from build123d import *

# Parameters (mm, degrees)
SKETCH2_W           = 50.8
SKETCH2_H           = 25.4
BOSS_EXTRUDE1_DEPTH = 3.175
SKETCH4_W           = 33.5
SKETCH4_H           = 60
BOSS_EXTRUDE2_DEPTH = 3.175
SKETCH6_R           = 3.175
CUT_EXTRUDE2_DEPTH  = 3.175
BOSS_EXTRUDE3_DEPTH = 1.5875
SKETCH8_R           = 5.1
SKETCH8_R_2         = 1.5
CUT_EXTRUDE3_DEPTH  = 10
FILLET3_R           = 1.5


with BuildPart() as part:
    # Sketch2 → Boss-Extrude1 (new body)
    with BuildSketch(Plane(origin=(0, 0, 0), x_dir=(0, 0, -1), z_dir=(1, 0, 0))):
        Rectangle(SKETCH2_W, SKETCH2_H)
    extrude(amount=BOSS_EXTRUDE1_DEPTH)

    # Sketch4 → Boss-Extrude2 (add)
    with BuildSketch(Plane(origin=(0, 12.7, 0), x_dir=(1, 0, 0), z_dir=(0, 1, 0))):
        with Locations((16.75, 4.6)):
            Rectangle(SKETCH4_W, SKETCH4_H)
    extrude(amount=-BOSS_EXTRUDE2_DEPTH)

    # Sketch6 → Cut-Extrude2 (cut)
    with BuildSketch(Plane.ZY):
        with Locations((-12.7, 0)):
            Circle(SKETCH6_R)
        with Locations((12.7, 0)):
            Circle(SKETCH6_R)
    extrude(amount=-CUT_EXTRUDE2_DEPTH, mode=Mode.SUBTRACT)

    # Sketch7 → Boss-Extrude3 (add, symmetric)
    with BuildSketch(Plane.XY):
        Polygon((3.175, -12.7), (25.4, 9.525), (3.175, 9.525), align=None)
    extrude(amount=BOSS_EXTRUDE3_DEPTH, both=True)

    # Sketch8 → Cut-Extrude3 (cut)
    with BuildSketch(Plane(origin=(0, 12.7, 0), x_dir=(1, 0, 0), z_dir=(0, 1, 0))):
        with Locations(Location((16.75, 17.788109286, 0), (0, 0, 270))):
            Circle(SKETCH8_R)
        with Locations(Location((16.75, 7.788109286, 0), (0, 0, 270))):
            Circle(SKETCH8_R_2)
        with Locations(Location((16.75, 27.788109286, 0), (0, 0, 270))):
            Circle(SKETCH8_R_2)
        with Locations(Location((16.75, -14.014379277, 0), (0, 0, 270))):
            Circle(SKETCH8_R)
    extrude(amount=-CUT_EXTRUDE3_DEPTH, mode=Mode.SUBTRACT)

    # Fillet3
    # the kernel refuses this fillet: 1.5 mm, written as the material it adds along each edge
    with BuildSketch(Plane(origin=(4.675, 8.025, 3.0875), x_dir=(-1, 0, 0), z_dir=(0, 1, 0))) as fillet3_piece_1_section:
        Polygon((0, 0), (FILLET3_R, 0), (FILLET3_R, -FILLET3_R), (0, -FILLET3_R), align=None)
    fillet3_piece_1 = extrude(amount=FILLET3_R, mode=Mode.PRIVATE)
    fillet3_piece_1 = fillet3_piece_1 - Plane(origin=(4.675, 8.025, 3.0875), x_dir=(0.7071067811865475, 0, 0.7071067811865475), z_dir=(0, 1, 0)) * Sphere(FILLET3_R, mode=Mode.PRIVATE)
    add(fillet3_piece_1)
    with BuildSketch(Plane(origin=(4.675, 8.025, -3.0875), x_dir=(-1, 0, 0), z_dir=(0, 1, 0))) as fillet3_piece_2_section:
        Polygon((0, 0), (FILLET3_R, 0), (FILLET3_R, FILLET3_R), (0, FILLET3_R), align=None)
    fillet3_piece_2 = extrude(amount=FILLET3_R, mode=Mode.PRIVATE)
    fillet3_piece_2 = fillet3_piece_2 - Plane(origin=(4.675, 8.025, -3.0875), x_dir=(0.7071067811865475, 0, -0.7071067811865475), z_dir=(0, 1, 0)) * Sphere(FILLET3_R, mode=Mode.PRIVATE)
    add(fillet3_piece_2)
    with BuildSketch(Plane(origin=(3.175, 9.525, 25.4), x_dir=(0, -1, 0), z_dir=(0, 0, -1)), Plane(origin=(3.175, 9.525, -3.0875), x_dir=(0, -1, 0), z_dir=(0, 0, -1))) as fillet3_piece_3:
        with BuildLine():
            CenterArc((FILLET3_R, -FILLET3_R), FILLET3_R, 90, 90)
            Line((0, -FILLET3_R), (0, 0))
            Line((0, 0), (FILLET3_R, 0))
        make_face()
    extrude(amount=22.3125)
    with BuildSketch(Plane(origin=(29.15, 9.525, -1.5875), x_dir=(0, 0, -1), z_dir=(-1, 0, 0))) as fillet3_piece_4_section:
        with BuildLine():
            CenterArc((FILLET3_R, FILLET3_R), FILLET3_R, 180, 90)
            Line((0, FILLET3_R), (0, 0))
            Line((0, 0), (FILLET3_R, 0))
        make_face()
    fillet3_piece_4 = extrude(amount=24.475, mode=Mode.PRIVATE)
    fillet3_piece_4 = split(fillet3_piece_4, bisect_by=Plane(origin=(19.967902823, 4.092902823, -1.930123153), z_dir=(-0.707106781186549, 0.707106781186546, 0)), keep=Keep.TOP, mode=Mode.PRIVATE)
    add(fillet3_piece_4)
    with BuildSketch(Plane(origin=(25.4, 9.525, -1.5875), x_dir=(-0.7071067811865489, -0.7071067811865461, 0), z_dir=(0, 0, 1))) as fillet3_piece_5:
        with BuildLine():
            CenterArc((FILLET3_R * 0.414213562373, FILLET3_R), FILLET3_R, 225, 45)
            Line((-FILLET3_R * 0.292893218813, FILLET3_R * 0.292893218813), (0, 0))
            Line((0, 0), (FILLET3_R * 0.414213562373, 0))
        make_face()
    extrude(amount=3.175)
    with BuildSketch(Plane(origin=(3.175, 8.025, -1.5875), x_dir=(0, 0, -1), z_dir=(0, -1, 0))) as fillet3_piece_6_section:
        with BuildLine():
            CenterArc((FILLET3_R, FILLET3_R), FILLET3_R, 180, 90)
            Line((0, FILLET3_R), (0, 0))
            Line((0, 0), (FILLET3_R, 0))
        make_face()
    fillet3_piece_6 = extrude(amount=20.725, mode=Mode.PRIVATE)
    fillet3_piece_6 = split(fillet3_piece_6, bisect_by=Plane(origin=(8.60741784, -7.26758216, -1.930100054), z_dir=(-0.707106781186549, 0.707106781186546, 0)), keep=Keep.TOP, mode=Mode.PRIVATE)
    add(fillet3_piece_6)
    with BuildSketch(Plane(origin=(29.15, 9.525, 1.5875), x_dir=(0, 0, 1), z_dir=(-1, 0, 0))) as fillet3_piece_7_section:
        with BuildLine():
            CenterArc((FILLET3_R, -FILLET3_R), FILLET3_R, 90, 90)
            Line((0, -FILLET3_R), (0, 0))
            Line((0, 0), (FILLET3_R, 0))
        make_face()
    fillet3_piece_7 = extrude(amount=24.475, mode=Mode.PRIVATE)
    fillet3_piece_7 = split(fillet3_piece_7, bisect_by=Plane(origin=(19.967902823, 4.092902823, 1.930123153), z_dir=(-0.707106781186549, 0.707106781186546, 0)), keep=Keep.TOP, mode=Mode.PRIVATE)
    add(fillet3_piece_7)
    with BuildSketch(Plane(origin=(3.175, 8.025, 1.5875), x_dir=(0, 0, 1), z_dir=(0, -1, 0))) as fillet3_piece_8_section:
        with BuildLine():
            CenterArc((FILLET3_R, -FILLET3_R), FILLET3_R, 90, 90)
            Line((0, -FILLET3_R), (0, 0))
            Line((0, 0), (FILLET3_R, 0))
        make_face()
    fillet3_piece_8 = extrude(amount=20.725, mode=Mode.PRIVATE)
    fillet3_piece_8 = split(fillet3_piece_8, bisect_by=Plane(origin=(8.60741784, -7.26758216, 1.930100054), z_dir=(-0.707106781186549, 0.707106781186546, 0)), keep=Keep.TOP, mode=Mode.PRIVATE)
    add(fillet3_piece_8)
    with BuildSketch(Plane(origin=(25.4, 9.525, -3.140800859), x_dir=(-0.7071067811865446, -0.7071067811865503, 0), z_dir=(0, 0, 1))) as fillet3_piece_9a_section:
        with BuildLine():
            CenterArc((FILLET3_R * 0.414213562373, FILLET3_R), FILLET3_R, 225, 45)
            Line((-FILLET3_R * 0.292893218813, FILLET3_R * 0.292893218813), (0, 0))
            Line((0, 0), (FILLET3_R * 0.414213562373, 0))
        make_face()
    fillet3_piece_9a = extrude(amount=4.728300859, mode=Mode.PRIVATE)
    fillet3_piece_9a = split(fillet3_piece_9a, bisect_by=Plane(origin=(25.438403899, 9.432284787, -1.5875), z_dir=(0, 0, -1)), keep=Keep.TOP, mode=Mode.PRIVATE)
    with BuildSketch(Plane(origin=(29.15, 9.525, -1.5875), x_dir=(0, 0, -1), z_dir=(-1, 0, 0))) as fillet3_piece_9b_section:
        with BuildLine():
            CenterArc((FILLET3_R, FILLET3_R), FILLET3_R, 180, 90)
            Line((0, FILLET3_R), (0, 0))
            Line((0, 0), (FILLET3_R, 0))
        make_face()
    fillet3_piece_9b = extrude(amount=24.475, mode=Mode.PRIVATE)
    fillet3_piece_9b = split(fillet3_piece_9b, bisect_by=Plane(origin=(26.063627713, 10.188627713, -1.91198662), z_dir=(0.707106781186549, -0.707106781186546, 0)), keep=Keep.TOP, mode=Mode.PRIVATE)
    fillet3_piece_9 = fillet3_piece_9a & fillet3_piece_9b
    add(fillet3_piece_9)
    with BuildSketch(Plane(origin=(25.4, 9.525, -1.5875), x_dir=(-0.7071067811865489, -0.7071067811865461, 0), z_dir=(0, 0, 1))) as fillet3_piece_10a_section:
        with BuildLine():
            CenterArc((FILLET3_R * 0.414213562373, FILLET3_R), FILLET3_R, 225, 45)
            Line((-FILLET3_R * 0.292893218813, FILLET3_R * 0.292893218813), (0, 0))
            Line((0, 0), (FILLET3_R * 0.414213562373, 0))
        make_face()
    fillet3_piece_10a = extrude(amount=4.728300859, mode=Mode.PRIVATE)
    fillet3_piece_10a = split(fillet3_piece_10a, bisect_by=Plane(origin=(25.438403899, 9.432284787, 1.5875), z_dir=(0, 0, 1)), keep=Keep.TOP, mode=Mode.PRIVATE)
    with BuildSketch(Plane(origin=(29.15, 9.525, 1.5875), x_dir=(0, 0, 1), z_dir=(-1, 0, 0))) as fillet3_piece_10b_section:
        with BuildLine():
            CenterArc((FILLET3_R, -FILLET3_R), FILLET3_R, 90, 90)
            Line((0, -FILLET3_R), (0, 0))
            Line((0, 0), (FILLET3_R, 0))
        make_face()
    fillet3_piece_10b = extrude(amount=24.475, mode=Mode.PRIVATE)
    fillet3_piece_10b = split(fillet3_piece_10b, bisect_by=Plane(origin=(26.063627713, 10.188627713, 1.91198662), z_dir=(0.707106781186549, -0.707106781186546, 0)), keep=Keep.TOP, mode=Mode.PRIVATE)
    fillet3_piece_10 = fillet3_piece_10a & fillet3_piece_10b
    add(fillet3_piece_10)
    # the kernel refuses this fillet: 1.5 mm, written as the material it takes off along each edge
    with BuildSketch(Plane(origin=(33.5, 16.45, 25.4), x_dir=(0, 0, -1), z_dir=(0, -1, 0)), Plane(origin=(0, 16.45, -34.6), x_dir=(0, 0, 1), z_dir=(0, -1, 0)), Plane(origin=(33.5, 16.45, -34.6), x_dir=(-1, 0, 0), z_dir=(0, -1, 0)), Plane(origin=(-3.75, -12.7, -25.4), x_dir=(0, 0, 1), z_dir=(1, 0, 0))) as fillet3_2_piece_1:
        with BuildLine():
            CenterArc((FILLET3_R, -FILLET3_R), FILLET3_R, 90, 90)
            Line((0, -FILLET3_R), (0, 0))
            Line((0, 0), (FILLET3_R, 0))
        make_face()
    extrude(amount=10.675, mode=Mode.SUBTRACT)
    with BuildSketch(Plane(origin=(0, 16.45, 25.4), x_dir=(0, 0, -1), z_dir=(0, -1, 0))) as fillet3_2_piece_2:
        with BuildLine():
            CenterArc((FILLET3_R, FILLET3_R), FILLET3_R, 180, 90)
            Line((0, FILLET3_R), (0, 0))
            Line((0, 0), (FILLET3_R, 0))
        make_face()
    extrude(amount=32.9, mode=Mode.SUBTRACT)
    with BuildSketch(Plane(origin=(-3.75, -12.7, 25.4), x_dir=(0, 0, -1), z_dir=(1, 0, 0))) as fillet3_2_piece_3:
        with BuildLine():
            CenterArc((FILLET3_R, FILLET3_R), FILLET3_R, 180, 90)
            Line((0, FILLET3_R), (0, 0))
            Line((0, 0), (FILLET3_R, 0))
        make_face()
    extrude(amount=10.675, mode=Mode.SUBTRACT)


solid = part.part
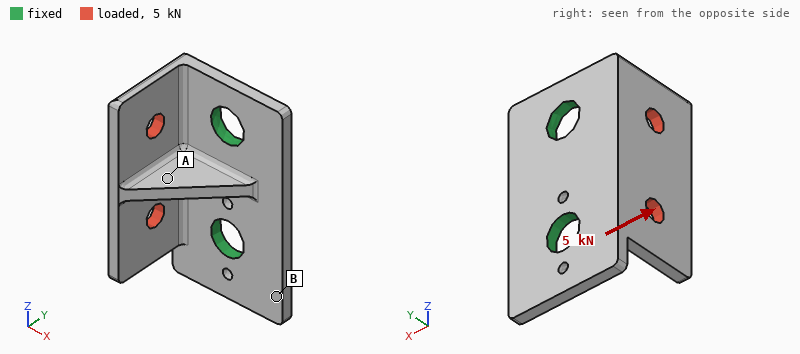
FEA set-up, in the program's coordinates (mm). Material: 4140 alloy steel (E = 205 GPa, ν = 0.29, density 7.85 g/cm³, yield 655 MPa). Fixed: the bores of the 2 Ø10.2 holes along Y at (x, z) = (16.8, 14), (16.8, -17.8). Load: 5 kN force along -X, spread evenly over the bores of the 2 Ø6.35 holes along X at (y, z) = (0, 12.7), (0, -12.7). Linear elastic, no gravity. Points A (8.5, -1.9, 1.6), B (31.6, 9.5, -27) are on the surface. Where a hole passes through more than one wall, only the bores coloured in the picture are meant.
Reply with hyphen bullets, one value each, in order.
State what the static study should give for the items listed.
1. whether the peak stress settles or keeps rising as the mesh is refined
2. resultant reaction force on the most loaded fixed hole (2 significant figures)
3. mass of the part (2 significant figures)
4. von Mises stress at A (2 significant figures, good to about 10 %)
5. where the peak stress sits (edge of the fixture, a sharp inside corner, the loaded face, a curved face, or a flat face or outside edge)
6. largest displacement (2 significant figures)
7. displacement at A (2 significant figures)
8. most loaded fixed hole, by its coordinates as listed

- keeps rising
- 2.8 kN
- 79 g
- 110 MPa
- edge of the fixture
- 0.23 mm
- 0.076 mm
- (16.8, 14)
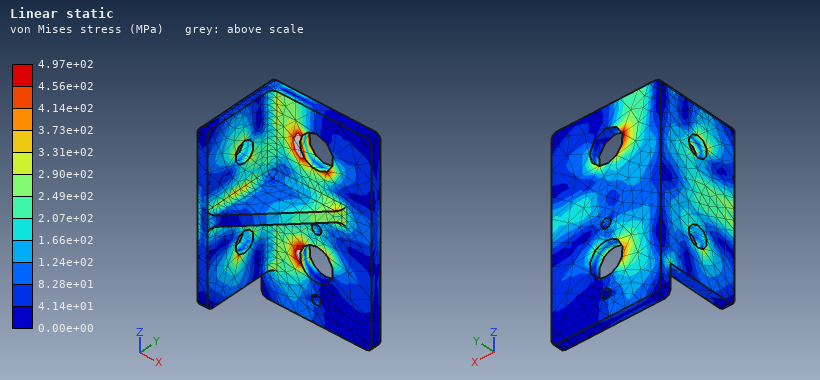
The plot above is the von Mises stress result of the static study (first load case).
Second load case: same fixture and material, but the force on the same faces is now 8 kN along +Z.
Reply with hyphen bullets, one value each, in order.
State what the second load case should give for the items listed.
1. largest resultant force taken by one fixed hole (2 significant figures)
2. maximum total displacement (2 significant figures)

- 5.5 kN
- 0.14 mm
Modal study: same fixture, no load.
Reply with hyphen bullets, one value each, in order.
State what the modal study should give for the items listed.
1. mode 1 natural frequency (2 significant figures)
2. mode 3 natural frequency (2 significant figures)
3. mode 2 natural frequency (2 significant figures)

- 4600 Hz
- 8400 Hz
- 5600 Hz
